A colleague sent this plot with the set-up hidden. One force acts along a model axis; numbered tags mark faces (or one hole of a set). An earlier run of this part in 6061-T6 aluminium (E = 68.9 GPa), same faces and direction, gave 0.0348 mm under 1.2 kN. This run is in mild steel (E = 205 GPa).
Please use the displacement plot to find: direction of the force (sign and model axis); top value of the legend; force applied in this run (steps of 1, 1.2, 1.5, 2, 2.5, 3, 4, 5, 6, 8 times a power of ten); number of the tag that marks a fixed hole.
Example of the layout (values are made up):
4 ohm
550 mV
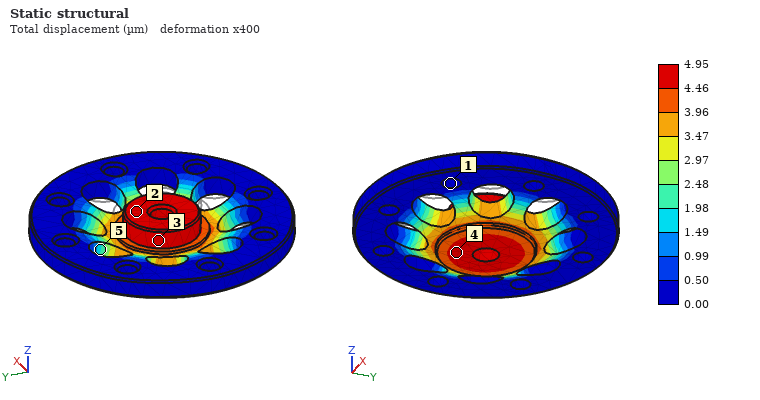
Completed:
-Z
4.95 µm
500 N
1
